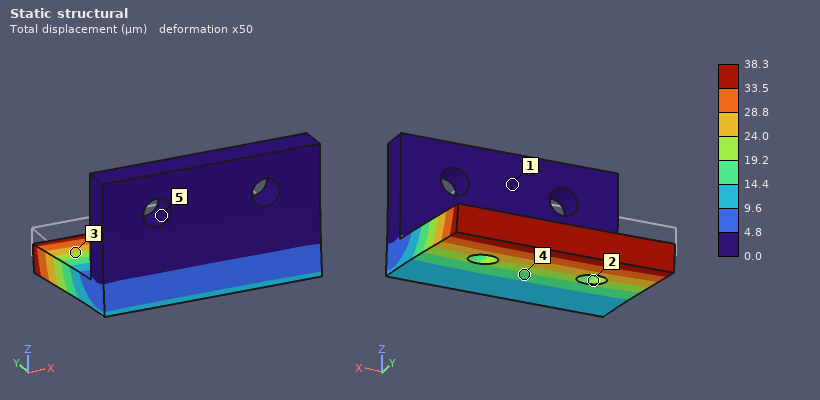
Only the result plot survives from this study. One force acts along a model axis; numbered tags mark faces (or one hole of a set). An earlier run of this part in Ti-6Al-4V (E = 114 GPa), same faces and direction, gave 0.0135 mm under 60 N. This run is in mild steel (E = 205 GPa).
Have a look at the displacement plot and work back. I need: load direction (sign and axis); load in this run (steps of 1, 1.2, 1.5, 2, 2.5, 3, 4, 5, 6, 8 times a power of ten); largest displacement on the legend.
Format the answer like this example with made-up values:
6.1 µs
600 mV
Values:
-Z
300 N
38.3 µm
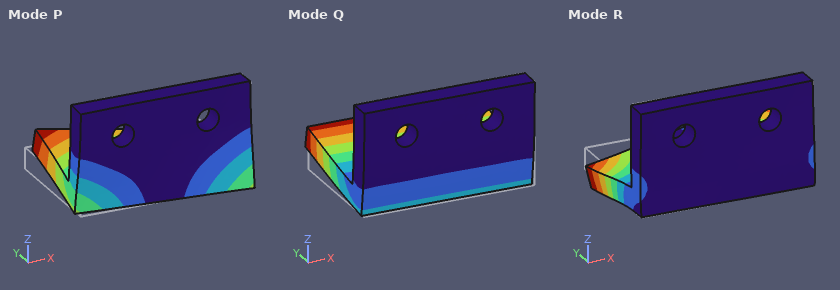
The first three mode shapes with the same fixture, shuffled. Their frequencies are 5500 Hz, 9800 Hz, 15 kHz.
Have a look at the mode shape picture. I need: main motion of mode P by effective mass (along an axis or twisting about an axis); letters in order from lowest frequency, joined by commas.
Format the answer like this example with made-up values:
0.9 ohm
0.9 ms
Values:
along X
Q, P, R
